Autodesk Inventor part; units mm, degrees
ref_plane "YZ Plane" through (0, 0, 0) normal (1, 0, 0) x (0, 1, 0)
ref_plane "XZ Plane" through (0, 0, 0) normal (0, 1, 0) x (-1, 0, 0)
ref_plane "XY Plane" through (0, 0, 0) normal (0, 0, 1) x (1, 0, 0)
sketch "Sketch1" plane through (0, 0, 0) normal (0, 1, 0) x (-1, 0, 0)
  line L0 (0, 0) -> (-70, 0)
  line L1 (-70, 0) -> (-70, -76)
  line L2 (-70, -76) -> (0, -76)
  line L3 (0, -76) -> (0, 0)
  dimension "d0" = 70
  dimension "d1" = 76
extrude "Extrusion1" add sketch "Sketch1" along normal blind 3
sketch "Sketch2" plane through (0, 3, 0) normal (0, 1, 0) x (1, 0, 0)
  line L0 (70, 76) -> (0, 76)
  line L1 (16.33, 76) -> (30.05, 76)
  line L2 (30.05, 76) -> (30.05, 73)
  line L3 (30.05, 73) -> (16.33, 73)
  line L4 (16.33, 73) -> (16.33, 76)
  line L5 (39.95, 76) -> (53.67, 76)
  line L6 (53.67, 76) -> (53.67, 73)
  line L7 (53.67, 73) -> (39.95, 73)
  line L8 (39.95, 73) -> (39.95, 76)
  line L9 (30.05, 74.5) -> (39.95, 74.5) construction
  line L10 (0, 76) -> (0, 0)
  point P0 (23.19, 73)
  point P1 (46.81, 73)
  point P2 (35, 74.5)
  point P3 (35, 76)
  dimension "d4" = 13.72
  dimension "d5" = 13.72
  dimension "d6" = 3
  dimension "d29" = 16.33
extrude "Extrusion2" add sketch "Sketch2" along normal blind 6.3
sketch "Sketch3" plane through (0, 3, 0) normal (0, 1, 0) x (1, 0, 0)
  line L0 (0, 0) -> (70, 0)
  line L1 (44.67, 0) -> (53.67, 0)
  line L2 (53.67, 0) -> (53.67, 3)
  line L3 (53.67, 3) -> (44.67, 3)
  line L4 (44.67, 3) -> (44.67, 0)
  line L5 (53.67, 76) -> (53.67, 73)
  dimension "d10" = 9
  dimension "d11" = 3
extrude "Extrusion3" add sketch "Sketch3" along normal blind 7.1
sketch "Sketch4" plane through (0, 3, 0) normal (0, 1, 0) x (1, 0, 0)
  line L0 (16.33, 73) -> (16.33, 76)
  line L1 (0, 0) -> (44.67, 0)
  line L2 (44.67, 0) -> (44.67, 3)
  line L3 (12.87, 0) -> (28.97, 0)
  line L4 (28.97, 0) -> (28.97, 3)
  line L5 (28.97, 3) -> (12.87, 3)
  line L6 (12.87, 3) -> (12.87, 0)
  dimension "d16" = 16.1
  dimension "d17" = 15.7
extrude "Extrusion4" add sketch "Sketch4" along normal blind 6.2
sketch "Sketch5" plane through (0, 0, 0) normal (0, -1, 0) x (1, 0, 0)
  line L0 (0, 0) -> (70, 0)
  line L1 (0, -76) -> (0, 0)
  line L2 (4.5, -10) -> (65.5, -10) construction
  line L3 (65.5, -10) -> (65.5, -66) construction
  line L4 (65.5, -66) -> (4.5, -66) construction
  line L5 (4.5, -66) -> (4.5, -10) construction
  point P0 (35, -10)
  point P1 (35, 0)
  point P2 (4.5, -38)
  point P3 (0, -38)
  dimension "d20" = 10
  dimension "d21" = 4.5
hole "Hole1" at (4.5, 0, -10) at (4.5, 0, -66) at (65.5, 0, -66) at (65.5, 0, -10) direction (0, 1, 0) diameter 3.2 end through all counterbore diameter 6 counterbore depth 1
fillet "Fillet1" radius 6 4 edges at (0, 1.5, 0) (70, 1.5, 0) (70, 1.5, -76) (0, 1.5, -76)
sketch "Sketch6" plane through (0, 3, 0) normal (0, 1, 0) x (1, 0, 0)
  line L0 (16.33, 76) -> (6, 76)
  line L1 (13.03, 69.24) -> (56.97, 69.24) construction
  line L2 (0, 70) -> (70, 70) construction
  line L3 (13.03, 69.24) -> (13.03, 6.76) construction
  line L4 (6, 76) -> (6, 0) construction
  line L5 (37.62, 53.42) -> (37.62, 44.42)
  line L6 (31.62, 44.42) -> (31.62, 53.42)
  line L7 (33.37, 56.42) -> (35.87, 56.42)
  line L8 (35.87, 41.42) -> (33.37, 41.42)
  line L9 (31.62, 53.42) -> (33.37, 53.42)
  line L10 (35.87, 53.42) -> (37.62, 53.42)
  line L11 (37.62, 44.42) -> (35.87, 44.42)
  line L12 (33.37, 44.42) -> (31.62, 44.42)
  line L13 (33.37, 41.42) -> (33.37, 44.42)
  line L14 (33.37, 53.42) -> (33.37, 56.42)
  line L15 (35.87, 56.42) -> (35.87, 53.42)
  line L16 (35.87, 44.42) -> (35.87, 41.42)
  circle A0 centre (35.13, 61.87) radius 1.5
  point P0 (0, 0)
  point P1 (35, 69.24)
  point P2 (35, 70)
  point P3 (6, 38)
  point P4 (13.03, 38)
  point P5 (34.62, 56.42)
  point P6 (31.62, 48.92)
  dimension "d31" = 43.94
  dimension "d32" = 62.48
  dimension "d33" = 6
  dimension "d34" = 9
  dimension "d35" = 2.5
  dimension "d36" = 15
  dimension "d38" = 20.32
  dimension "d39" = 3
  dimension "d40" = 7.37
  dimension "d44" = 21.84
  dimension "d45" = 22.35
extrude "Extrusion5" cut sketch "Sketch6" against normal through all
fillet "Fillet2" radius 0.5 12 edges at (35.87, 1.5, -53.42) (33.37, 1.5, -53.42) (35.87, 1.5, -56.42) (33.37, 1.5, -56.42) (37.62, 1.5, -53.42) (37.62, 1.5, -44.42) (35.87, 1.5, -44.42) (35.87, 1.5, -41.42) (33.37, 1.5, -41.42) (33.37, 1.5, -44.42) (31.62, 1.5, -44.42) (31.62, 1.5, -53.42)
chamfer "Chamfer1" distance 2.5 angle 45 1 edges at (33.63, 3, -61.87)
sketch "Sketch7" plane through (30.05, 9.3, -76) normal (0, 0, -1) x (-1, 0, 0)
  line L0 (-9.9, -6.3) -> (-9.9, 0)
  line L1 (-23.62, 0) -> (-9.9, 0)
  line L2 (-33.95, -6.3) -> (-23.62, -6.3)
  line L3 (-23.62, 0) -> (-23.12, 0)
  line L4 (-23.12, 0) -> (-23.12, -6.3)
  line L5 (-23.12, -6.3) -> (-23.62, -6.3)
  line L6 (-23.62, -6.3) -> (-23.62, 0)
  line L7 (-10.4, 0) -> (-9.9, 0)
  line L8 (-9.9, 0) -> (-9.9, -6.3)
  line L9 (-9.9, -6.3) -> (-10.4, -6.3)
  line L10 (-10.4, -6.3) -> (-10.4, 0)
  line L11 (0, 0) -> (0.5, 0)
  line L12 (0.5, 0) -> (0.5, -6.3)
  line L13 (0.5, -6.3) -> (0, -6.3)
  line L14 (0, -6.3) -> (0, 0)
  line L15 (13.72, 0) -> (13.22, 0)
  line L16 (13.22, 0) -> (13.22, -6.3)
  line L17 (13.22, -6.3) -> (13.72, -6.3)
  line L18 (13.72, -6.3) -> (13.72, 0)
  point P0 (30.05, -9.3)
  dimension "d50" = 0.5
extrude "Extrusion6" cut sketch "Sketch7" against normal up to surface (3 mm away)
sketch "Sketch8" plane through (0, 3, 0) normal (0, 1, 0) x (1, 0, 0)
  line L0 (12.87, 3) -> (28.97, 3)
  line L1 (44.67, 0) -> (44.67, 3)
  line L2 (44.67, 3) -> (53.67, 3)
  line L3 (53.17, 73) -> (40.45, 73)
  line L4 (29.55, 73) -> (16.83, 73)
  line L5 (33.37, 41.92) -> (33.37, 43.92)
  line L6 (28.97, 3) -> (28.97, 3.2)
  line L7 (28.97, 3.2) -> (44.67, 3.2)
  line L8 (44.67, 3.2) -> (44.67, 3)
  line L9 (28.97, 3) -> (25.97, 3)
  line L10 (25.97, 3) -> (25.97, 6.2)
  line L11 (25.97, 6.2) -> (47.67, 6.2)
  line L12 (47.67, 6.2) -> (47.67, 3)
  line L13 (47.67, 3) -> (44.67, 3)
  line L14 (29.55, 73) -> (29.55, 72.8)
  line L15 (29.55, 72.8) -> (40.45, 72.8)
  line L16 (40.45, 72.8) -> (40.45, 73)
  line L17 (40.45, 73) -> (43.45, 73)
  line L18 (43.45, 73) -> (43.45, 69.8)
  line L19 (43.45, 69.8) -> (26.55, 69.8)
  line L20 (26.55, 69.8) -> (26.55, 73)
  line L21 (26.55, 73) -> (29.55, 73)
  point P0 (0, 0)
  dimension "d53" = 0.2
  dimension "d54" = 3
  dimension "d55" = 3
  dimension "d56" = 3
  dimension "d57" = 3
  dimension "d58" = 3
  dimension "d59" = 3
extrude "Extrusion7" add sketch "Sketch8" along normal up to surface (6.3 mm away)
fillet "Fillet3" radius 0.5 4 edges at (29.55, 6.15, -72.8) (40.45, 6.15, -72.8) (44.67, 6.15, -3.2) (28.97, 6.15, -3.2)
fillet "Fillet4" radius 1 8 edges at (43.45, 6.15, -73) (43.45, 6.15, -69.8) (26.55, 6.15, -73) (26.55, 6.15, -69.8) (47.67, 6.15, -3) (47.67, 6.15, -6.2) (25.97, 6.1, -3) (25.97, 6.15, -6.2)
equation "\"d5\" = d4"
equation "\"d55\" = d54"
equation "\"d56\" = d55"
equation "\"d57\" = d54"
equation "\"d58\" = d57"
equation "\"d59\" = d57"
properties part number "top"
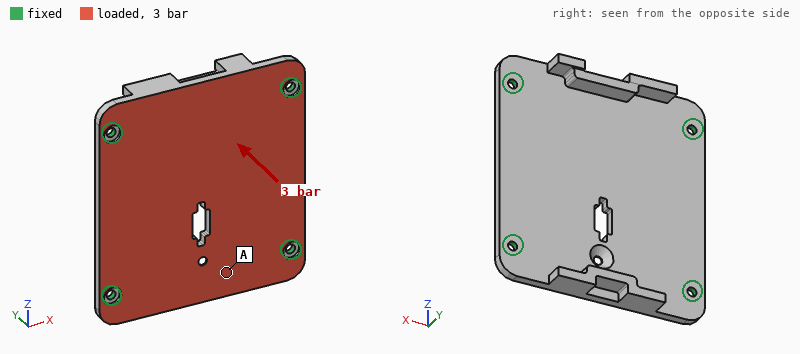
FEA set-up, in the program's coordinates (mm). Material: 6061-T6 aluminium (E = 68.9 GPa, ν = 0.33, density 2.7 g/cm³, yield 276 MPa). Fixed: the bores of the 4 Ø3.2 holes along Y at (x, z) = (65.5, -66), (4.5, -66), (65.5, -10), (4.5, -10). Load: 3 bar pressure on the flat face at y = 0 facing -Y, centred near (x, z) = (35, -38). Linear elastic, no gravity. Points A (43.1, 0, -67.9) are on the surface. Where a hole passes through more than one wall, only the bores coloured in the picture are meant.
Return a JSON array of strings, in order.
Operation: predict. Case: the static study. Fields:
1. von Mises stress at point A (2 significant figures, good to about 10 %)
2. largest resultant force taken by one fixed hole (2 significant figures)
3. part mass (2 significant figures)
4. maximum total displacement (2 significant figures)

["30 MPa", "470 N", "46 g", "0.18 mm"]
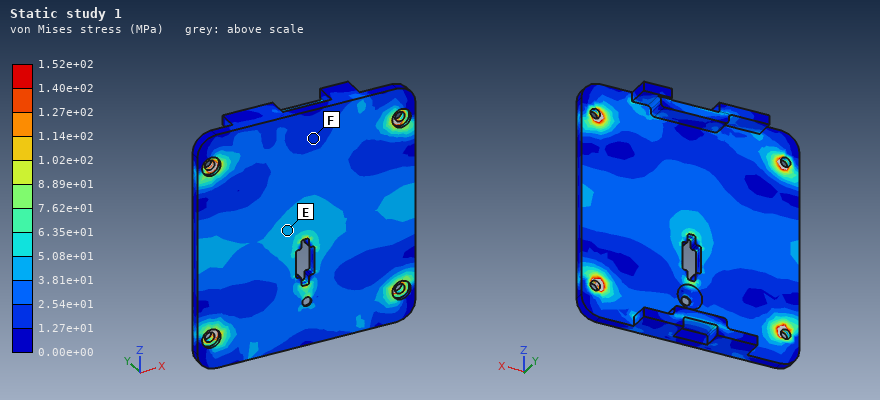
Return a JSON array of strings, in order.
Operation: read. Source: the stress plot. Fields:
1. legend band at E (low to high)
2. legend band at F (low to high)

["3.81e+01 to 5.08e+01 MPa", "1.27e+01 to 2.54e+01 MPa"]
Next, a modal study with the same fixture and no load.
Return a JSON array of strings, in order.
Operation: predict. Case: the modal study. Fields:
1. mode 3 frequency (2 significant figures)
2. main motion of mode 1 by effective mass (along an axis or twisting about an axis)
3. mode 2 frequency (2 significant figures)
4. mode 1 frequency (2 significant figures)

["4400 Hz", "along Y", "4300 Hz", "2800 Hz"]
